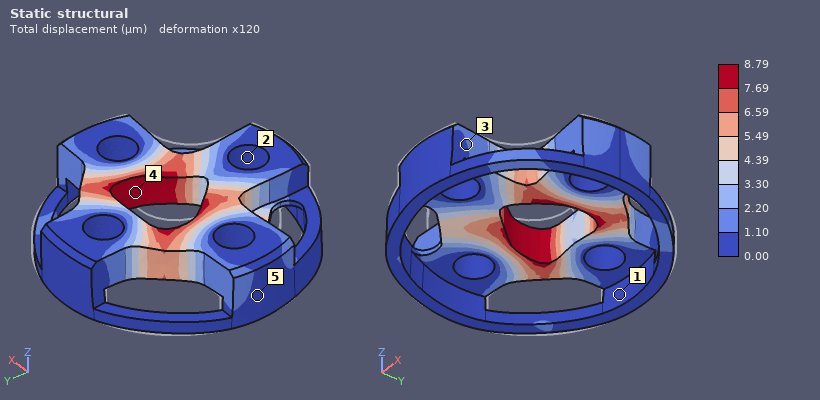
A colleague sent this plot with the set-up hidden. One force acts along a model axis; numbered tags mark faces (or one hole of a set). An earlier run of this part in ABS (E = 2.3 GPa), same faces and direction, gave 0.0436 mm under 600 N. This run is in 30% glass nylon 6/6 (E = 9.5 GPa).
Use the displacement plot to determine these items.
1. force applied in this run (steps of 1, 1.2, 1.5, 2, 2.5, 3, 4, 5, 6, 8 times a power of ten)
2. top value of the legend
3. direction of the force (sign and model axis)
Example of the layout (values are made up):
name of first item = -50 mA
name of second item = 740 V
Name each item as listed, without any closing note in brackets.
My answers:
force applied in this run = 500 N
top value of the legend = 8.79 µm
direction of the force = +Y
